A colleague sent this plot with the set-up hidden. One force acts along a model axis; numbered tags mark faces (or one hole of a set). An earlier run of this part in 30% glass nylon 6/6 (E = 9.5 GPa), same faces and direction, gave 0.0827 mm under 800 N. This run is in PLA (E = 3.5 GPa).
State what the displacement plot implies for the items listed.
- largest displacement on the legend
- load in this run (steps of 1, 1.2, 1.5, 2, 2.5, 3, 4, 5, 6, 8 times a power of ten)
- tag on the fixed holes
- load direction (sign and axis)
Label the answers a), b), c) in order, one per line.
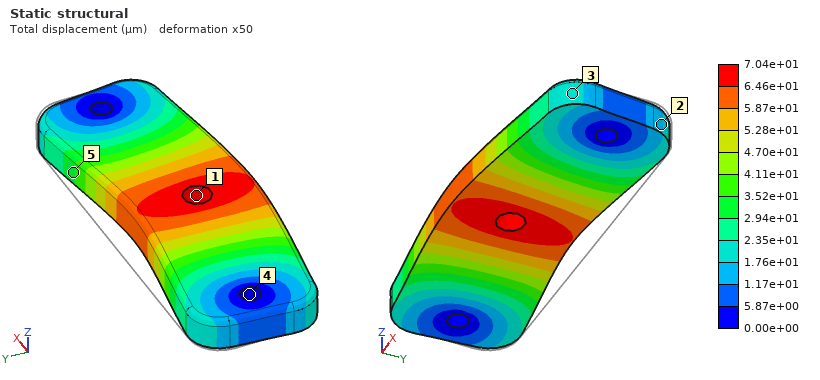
a) 7.04e+01 µm
b) 250 N
c) 4
d) -Y
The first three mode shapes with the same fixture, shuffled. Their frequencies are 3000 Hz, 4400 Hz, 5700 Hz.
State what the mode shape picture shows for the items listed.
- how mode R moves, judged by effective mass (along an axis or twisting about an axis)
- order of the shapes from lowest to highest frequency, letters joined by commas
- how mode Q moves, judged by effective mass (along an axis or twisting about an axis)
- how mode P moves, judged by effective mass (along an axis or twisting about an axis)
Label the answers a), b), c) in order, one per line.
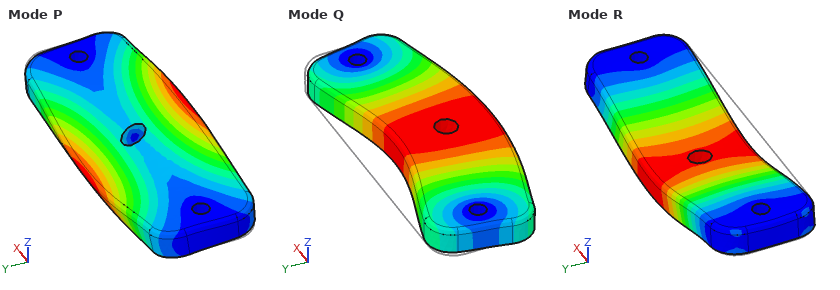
a) along Z
b) R, P, Q
c) along Y
d) twisting about X
